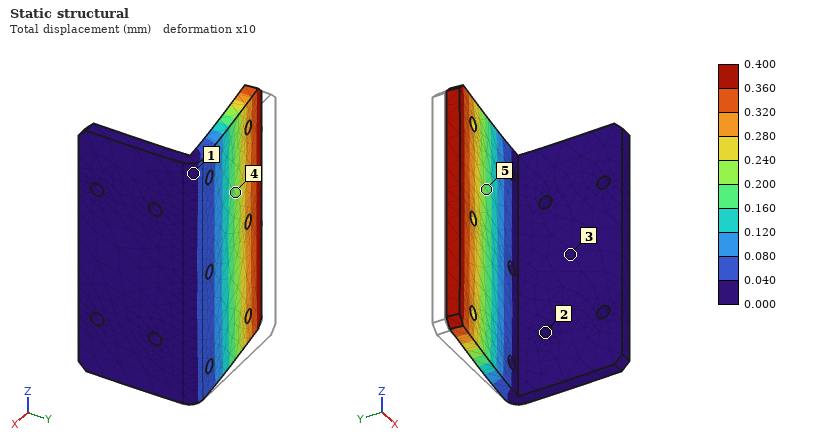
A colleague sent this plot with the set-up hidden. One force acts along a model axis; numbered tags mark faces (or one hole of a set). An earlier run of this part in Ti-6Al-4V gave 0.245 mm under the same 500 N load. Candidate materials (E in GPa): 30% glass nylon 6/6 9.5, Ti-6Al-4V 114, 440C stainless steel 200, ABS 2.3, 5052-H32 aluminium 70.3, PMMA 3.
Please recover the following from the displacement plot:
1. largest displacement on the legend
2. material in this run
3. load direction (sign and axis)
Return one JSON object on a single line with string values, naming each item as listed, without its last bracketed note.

{"largest displacement on the legend": "0.400 mm", "material in this run": "5052-H32 aluminium", "load direction": "-Y"}
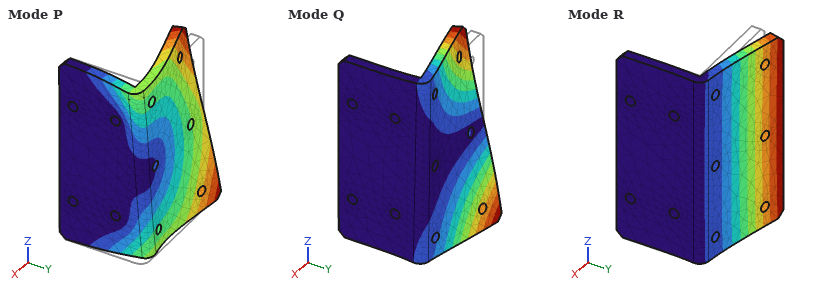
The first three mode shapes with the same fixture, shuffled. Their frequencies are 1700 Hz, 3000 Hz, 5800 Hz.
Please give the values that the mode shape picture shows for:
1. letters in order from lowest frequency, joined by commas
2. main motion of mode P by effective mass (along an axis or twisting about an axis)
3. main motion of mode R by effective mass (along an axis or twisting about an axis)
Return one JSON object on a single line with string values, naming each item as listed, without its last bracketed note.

{"letters in order from lowest frequency, joined by commas": "R, Q, P", "main motion of mode P by effective mass": "along Z", "main motion of mode R by effective mass": "along Y"}
